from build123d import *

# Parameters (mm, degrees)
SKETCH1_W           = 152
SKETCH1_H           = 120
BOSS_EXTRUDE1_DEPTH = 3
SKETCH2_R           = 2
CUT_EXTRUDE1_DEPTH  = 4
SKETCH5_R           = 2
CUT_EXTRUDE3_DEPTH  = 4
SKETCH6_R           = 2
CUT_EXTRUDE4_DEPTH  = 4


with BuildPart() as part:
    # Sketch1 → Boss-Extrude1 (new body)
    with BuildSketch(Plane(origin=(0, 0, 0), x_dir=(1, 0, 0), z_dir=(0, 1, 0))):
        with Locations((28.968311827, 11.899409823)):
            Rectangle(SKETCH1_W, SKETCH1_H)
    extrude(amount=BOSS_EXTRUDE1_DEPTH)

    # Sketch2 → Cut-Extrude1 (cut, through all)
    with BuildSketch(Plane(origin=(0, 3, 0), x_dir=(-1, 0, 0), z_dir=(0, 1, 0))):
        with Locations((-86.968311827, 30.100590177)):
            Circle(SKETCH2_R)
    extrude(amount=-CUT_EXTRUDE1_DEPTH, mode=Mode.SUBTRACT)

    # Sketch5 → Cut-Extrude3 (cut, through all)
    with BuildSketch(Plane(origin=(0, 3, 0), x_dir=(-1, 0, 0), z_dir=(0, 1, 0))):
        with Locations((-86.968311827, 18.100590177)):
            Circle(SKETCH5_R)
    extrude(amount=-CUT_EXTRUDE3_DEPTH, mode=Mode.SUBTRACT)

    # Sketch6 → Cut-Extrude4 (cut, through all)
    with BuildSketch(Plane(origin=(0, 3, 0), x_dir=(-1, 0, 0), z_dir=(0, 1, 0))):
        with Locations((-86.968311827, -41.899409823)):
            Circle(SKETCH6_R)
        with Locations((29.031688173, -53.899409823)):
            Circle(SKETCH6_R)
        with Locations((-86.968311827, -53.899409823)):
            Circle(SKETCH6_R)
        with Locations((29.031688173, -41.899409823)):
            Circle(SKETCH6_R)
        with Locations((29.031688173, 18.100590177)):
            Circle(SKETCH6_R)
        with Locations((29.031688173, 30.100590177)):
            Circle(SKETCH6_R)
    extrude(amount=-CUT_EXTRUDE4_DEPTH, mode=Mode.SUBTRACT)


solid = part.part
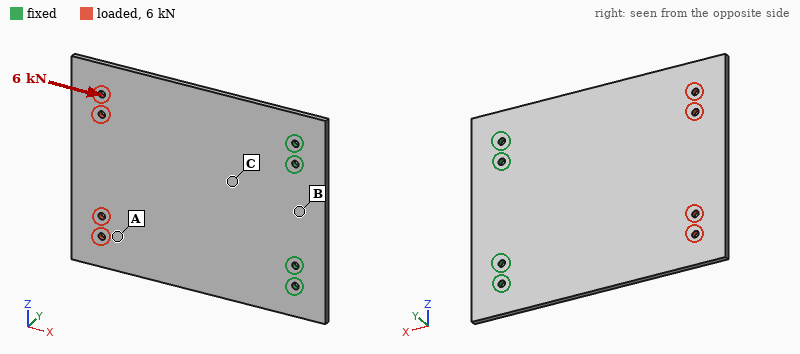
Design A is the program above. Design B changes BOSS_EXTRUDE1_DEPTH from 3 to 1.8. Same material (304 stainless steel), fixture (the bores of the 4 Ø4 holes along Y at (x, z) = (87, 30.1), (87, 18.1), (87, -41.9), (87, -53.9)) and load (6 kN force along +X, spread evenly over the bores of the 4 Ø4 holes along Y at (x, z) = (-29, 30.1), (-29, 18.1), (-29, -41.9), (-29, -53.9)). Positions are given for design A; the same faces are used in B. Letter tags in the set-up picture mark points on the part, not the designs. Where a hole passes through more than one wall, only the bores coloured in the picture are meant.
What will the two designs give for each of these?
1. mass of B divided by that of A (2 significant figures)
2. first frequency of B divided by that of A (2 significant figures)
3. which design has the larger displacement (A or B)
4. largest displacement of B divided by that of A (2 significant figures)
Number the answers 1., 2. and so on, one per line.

1. 0.60
2. 0.60
3. B
4. 1.7
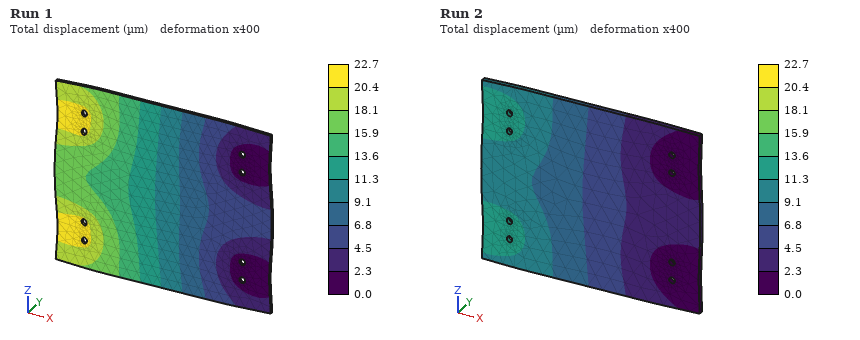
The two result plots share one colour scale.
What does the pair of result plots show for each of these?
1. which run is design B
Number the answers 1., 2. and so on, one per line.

1. Run 1
